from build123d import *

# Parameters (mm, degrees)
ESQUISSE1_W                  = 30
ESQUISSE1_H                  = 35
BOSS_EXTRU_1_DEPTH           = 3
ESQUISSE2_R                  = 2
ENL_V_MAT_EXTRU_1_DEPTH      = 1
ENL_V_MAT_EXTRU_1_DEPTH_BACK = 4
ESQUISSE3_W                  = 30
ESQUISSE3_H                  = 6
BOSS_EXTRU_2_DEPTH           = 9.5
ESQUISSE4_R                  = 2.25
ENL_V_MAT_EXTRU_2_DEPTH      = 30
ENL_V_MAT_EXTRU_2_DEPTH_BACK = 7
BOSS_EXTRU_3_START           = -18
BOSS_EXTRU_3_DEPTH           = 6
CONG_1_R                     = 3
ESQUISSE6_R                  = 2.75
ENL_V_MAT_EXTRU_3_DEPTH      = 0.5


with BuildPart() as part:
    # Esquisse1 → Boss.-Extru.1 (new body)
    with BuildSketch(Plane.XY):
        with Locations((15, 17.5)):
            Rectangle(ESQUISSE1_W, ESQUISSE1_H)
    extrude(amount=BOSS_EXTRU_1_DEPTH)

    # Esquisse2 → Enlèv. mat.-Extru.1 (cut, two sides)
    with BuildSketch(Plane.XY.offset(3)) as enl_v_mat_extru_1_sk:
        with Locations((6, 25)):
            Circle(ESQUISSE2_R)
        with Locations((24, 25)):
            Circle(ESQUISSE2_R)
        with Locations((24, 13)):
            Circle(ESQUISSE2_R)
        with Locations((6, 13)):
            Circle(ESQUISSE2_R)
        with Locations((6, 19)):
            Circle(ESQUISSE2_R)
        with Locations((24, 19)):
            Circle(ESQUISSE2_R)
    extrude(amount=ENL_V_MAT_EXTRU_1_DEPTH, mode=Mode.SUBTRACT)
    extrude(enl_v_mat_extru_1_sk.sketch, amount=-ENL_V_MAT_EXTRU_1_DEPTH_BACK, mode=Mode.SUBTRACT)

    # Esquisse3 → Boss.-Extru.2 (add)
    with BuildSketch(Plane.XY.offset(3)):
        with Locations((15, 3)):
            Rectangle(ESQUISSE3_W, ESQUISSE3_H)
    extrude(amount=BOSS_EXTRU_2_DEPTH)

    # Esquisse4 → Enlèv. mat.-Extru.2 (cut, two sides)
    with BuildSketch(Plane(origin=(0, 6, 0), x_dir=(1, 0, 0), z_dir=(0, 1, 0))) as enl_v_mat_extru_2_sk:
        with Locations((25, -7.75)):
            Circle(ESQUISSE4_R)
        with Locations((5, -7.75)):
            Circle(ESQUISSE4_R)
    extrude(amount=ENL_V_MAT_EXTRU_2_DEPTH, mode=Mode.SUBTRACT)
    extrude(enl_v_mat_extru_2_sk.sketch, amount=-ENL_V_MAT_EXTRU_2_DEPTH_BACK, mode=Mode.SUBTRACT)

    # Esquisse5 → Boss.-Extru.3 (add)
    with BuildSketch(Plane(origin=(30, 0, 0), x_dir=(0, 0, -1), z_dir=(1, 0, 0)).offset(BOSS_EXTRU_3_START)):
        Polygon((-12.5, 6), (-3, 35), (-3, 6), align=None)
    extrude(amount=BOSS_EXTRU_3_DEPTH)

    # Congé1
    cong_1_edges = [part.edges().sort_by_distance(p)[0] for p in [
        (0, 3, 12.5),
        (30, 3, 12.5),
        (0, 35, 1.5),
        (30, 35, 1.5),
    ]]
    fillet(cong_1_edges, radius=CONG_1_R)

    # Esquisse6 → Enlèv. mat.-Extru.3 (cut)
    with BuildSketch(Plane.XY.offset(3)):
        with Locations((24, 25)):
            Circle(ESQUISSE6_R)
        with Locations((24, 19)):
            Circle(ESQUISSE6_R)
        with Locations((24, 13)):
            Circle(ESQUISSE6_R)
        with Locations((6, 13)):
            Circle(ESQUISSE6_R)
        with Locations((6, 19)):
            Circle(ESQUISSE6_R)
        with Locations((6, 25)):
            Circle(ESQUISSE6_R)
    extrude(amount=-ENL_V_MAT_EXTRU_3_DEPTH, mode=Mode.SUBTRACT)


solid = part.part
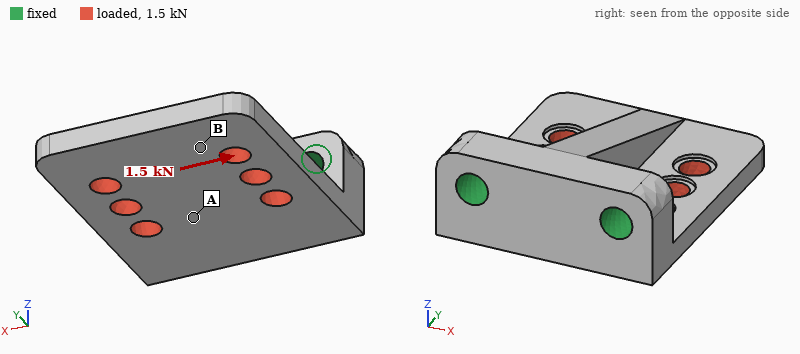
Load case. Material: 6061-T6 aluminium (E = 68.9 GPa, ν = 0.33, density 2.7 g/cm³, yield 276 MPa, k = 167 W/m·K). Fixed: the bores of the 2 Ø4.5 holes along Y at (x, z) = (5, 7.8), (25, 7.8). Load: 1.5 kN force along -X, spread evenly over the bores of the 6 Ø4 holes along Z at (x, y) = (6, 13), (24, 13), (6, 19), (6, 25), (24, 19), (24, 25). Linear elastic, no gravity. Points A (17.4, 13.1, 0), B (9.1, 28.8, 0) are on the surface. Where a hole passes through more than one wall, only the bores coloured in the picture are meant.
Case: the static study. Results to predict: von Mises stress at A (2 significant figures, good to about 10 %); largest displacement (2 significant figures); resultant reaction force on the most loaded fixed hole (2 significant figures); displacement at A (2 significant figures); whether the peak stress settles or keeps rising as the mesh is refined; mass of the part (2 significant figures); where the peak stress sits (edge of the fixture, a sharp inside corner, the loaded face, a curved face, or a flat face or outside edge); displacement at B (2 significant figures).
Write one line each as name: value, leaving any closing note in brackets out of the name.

von Mises stress at A: 46 MPa
largest displacement: 44 µm
resultant reaction force on the most loaded fixed hole: 1.4 kN
displacement at A: 13 µm
whether the peak stress settles or keeps rising as the mesh is refined: keeps rising
mass of the part: 14 g
where the peak stress sits: edge of the fixture
displacement at B: 37 µm
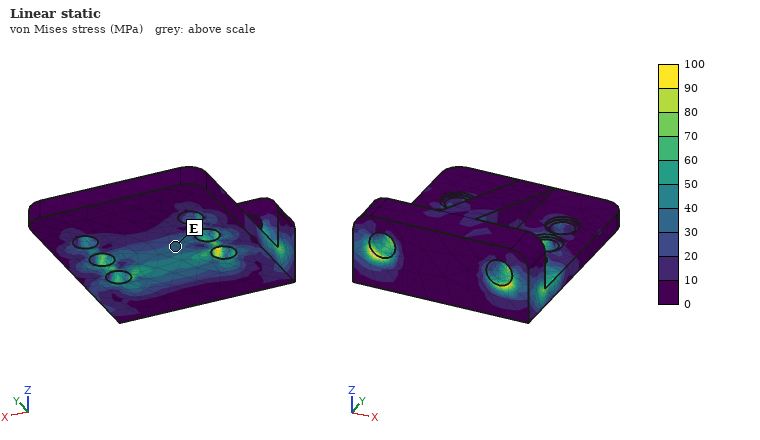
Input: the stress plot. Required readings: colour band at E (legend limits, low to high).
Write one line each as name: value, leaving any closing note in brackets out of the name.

colour band at E: 30 to 40 MPa
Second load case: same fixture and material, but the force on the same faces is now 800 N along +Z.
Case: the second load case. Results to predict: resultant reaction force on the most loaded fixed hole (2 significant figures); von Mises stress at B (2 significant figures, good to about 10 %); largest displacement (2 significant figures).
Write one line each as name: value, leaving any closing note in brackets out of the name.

resultant reaction force on the most loaded fixed hole: 410 N
von Mises stress at B: 23 MPa
largest displacement: 97 µm
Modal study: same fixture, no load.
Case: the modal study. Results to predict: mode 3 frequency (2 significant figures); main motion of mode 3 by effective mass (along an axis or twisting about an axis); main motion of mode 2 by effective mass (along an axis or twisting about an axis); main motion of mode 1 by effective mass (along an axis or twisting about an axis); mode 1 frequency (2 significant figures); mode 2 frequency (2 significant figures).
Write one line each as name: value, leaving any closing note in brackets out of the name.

mode 3 frequency: 12 kHz
main motion of mode 3 by effective mass: along X
main motion of mode 2 by effective mass: twisting about Y
main motion of mode 1 by effective mass: along Z
mode 1 frequency: 5900 Hz
mode 2 frequency: 8400 Hz
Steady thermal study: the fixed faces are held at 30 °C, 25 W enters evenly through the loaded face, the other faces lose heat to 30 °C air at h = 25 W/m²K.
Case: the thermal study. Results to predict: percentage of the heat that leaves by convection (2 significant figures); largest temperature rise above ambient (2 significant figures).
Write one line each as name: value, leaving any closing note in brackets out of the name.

percentage of the heat that leaves by convection: 4.1 %
largest temperature rise above ambient: 25 K
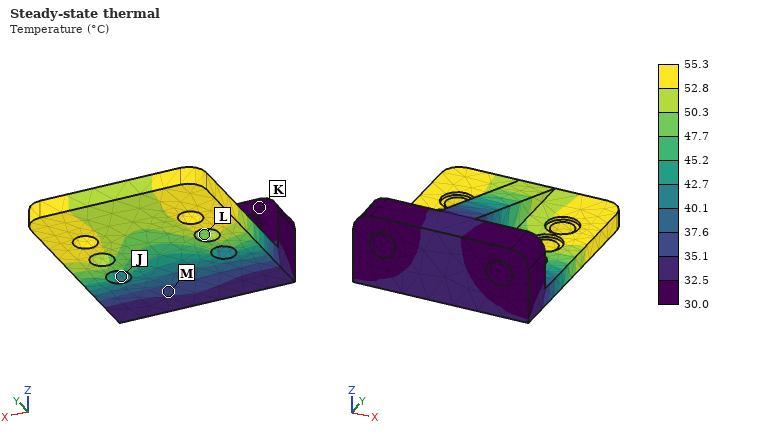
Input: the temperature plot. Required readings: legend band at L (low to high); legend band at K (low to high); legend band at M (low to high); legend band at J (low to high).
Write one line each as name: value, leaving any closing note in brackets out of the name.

legend band at L: 47.7 to 50.3 °C
legend band at K: 30.0 to 32.5 °C
legend band at M: 35.1 to 37.6 °C
legend band at J: 40.1 to 42.7 °C
